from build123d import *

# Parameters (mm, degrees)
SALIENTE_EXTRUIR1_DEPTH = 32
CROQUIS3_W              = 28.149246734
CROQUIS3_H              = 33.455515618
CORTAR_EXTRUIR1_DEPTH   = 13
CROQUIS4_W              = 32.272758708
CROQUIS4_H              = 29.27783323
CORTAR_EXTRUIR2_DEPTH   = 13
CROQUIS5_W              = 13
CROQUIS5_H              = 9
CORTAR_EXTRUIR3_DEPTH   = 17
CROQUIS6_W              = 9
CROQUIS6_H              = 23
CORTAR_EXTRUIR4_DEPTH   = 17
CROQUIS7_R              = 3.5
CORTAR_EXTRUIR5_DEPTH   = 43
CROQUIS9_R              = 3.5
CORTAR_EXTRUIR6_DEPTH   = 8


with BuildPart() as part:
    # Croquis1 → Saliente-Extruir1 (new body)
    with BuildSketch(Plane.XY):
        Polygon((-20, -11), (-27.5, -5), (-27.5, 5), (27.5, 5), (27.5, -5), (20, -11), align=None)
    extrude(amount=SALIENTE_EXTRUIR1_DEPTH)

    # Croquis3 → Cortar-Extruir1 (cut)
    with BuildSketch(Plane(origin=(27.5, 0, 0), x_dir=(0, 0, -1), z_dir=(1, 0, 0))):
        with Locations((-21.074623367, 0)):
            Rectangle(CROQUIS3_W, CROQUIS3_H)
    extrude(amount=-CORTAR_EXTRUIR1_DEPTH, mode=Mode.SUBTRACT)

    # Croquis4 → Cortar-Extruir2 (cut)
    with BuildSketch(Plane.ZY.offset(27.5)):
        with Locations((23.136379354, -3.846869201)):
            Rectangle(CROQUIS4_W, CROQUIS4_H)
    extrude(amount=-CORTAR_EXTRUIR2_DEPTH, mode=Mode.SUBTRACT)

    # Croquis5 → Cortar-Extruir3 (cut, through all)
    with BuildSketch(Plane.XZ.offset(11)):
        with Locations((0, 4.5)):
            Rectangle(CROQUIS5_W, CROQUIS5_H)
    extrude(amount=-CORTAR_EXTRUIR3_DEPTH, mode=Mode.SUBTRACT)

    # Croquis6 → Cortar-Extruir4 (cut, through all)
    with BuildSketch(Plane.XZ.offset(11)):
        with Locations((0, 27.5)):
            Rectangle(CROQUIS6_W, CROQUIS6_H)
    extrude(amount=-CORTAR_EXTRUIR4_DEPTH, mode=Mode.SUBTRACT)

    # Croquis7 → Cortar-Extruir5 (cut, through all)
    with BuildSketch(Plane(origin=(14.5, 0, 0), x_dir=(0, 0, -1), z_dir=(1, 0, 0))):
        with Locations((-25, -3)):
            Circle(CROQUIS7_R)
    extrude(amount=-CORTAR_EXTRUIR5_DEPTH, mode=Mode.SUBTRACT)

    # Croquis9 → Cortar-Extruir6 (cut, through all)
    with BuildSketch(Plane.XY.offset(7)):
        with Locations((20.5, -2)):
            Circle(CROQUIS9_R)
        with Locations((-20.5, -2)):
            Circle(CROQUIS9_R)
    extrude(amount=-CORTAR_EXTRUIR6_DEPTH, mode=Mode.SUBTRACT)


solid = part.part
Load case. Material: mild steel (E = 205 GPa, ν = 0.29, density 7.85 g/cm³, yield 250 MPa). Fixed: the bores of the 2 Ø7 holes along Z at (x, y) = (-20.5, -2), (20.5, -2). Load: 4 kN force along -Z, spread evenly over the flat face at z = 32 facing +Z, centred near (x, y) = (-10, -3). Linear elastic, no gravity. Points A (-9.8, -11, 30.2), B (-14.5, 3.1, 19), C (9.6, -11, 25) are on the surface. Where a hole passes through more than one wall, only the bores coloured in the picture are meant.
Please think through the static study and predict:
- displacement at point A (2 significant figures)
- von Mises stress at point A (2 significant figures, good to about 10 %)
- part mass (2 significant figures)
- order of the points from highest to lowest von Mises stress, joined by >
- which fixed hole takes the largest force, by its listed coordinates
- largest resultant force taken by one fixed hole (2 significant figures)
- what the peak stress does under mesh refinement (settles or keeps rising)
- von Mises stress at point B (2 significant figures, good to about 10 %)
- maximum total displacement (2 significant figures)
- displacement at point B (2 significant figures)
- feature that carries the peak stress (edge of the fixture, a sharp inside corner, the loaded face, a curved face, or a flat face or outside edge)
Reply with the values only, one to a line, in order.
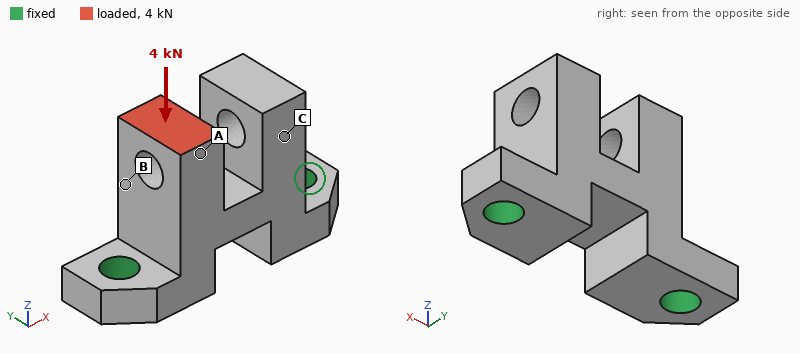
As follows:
8.6 µm
21 MPa
94 g
B > A > C
(-20.5, -2)
3.5 kN
keeps rising
36 MPa
11 µm
6.2 µm
edge of the fixture
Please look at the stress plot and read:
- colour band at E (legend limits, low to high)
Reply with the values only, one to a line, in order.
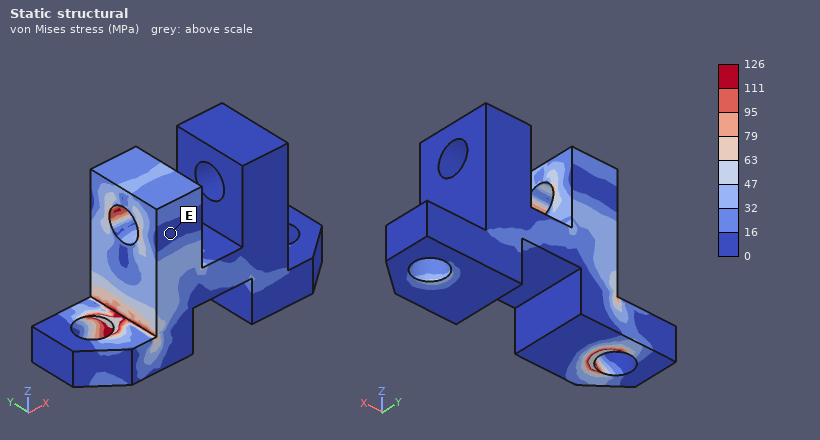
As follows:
0 to 16 MPa
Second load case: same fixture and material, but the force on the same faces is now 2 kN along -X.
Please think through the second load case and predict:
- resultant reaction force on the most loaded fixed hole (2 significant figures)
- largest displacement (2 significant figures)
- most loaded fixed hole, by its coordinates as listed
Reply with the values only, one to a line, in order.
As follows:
3.0 kN
43 µm
(20.5, -2)
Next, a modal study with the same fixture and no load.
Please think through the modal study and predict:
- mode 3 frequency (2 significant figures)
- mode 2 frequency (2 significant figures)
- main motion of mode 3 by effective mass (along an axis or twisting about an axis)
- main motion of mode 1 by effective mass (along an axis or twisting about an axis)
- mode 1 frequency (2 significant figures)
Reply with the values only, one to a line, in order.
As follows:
13 kHz
11 kHz
along X
along Y
6600 Hz
